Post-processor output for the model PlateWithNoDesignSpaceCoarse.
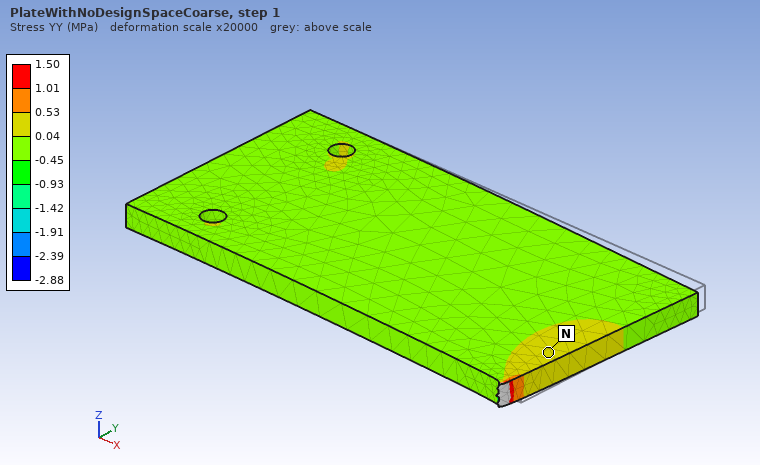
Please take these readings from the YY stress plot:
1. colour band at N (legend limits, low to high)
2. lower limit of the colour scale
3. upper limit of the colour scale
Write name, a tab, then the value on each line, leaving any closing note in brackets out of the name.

colour band at N	0.04 to 0.53 MPa
lower limit of the colour scale	-2.88 MPa
upper limit of the colour scale	1.50 MPa
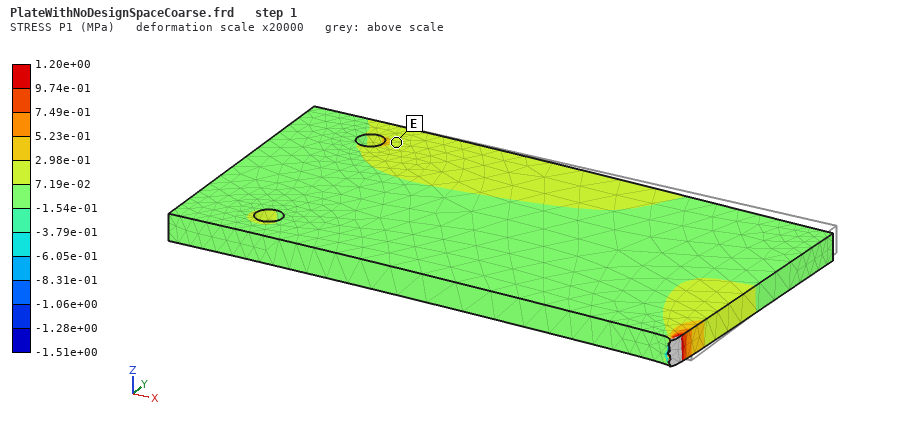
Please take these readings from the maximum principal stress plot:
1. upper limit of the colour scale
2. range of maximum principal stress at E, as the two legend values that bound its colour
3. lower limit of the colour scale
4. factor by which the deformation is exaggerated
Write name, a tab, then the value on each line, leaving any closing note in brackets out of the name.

upper limit of the colour scale	1.20e+00 MPa
range of maximum principal stress at E, as the two legend values that bound its colour	7.19e-02 to 2.98e-01 MPa
lower limit of the colour scale	-1.51e+00 MPa
factor by which the deformation is exaggerated	20000
